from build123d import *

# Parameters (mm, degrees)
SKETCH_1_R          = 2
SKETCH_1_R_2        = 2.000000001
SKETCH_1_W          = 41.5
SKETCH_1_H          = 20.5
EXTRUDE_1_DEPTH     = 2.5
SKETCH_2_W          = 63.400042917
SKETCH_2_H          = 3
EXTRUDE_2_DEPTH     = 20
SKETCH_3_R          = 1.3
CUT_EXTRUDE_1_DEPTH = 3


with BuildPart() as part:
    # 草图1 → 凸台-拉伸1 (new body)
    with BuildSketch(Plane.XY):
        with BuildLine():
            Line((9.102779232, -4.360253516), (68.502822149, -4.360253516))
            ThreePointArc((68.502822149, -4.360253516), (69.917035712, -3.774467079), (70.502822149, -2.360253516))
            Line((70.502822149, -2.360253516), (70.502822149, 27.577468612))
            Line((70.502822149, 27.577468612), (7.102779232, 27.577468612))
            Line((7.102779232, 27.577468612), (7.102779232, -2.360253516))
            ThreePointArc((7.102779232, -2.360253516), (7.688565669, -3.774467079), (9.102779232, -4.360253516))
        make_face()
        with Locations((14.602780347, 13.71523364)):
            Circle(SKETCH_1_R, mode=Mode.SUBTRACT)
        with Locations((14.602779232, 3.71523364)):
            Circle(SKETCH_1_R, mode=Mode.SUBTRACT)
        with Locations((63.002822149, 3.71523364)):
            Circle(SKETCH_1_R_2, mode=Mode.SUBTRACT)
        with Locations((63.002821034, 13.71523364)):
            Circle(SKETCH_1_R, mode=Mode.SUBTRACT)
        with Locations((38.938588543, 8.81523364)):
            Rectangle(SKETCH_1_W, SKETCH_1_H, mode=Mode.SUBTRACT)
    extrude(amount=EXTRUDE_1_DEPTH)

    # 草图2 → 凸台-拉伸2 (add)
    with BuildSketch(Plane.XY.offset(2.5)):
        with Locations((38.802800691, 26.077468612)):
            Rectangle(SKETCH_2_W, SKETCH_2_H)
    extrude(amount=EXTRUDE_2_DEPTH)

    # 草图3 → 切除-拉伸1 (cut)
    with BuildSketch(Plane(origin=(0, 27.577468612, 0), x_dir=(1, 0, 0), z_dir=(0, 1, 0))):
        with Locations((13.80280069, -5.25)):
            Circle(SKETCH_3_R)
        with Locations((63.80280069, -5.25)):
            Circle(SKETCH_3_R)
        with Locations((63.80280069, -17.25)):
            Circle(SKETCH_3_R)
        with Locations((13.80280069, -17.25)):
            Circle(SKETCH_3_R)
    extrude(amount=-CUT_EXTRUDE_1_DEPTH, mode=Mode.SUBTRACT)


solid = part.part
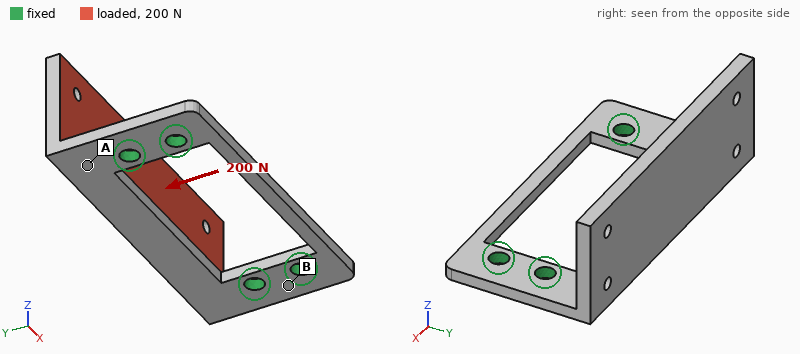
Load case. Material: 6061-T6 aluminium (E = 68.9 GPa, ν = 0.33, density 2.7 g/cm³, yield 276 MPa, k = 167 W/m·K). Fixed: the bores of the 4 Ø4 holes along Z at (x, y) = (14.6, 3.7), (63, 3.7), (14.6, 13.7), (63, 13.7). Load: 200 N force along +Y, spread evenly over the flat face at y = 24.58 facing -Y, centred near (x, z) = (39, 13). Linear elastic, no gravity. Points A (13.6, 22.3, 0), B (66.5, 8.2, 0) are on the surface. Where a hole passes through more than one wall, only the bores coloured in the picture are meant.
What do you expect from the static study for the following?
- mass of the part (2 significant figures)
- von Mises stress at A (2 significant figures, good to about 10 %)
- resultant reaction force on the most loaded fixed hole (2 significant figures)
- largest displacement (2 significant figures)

18 g
65 MPa
110 N
0.29 mm
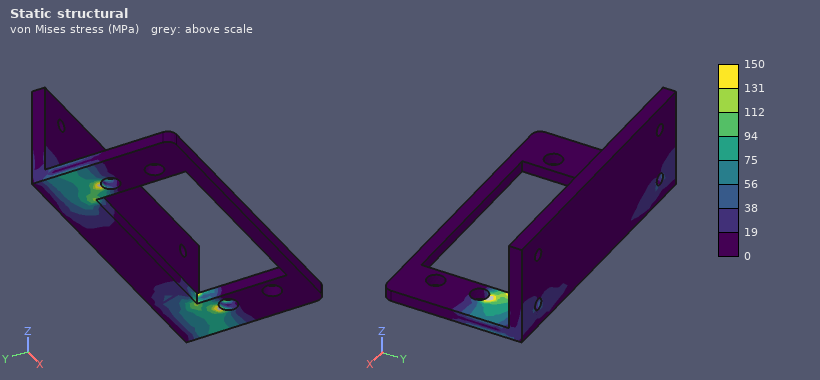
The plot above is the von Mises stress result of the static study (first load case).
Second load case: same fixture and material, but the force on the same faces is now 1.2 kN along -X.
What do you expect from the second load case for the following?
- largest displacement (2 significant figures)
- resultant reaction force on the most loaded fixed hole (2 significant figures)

0.17 mm
790 N
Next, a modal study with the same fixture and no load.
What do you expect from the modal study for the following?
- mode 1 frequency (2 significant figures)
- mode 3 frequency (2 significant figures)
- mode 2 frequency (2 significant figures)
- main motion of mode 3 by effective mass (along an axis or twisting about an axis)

1500 Hz
5300 Hz
3700 Hz
along Z
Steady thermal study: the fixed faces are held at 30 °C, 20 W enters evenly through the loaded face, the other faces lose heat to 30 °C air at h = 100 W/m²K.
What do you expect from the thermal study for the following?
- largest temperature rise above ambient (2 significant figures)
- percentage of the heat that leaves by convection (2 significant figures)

25 K
29 %
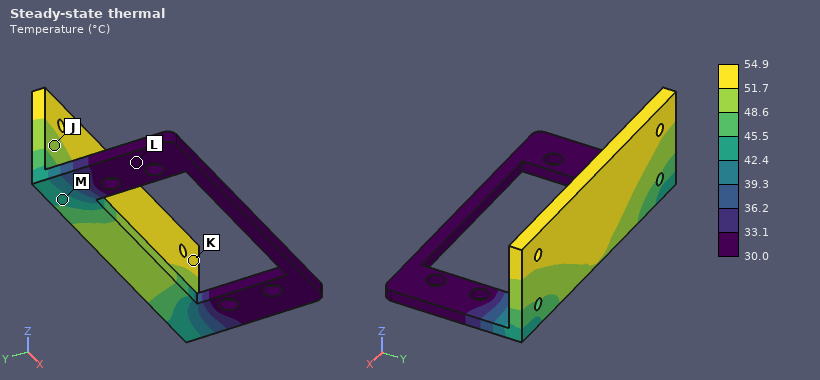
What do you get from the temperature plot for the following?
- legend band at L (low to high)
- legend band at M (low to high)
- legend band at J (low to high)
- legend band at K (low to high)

30.0 to 33.1 °C
42.4 to 45.5 °C
48.6 to 51.7 °C
51.7 to 54.9 °C
